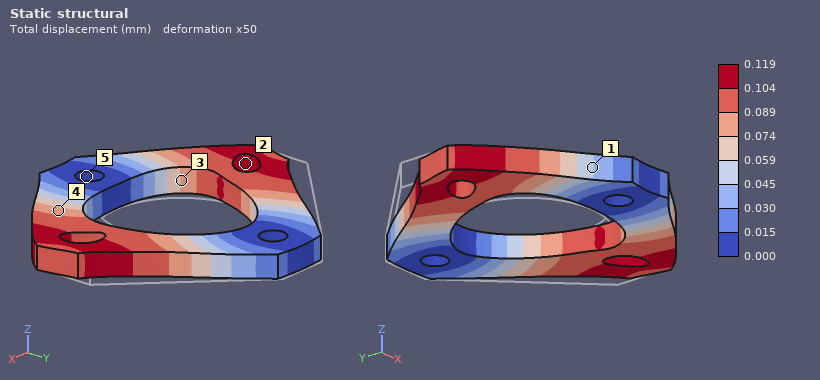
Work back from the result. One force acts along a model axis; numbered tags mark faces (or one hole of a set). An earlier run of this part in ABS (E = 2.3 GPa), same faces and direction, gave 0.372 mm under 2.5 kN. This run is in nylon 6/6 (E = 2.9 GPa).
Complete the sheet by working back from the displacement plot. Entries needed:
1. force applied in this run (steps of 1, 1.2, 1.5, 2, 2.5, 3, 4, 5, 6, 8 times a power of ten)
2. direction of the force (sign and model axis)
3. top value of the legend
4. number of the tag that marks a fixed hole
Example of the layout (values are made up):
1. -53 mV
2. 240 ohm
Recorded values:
1. 1 kN
2. -Y
3. 0.119 mm
4. 5
